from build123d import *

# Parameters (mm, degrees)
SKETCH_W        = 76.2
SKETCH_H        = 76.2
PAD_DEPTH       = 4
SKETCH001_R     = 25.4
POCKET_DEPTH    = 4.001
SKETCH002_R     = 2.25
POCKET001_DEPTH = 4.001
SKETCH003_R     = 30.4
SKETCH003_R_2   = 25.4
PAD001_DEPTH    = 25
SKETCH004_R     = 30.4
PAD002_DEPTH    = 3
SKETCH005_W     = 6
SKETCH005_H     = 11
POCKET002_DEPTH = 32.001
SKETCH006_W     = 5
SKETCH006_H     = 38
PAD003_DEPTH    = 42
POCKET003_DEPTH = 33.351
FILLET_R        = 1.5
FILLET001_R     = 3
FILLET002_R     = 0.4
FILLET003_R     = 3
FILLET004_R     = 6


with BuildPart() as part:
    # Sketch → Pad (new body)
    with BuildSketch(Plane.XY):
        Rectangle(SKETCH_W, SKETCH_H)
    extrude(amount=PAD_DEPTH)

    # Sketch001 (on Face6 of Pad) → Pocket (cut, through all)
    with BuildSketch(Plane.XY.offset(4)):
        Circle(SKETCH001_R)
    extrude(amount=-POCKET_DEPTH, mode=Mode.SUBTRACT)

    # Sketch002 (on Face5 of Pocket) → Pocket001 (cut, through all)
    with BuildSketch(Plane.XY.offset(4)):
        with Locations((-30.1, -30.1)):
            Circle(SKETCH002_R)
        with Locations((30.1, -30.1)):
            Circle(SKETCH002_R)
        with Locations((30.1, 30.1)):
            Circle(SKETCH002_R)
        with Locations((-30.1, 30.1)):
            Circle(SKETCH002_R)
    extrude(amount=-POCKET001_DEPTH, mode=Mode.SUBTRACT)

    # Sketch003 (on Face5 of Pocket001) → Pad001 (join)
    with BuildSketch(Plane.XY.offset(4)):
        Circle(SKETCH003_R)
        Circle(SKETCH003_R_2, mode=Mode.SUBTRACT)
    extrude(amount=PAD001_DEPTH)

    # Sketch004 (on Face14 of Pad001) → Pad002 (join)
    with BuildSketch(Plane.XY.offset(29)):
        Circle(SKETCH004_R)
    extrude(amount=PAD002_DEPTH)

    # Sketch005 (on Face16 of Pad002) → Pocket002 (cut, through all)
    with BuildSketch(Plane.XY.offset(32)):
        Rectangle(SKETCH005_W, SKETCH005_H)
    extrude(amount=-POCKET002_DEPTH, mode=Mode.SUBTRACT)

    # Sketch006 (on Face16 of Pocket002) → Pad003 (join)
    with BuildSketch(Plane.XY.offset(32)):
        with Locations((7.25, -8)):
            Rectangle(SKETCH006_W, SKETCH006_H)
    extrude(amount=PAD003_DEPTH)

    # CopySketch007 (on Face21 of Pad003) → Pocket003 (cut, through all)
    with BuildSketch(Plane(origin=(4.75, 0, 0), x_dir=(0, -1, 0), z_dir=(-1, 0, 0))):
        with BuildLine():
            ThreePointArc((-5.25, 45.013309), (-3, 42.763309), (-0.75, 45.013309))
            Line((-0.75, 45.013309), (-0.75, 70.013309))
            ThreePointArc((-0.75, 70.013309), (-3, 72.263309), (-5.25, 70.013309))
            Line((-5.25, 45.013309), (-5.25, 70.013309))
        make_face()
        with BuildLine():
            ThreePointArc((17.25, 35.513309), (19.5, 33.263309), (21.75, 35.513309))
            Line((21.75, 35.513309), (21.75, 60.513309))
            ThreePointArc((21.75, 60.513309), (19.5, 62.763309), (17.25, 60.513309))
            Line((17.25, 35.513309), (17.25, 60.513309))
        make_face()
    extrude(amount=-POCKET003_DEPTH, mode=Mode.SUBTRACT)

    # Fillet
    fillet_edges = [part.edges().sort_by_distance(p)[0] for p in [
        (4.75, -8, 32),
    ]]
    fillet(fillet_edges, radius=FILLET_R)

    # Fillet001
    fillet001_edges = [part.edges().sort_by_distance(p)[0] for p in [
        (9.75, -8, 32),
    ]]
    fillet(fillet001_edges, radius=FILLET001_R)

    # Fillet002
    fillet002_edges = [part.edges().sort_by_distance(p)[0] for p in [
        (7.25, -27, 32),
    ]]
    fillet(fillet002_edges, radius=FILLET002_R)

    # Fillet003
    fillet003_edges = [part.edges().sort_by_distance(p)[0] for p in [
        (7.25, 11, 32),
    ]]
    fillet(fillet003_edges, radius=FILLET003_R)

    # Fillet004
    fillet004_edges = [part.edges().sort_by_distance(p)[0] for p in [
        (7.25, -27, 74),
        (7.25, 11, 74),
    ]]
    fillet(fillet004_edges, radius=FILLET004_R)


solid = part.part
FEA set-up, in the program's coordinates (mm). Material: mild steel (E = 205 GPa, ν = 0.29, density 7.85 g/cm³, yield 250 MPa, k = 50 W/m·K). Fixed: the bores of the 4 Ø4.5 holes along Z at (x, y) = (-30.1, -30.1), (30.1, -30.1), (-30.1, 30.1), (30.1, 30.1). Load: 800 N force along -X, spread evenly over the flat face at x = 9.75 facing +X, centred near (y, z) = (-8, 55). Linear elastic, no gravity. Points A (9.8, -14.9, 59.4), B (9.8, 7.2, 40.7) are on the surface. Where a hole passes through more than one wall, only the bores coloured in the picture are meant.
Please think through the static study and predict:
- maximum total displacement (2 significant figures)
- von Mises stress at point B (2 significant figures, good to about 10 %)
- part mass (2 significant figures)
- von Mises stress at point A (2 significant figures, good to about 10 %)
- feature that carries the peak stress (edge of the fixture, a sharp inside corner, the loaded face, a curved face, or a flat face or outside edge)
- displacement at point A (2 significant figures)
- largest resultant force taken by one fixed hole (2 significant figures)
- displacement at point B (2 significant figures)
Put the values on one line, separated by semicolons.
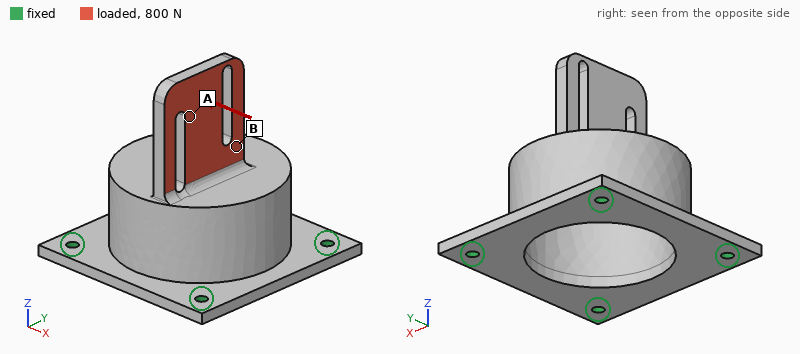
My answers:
0.19 mm; 78 MPa; 410 g; 24 MPa; a curved face; 0.12 mm; 470 N; 0.032 mm
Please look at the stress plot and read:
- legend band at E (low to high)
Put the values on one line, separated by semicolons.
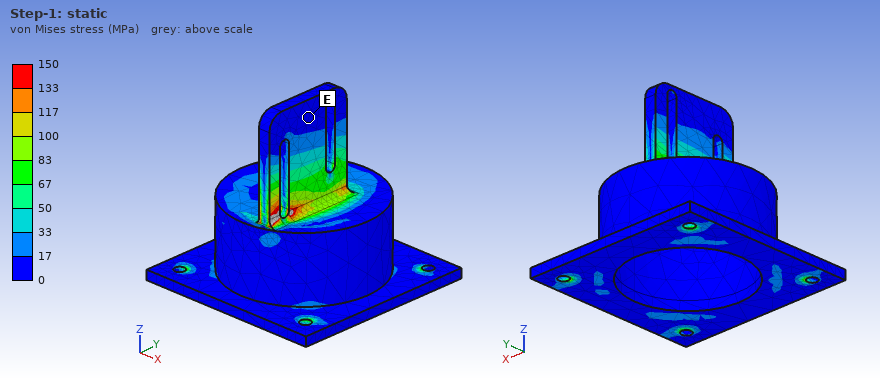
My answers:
0 to 17 MPa
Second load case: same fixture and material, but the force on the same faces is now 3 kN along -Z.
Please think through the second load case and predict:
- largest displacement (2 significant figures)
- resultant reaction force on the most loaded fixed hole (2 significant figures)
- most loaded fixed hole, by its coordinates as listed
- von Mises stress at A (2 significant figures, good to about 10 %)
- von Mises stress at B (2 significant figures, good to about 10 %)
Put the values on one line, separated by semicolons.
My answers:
81 µm; 1.3 kN; (30.1, -30.1); 25 MPa; 60 MPa
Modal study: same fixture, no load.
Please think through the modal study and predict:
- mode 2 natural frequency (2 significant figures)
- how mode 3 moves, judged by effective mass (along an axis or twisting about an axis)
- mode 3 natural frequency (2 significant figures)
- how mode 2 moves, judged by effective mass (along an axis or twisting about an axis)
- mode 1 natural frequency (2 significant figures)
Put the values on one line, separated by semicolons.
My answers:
3200 Hz; along Z; 4200 Hz; along Y; 1800 Hz
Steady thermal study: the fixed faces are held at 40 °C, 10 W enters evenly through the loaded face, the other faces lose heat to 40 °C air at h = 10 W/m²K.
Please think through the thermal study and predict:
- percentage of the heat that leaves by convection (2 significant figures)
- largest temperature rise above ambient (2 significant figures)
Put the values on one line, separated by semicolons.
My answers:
27 %; 47 K
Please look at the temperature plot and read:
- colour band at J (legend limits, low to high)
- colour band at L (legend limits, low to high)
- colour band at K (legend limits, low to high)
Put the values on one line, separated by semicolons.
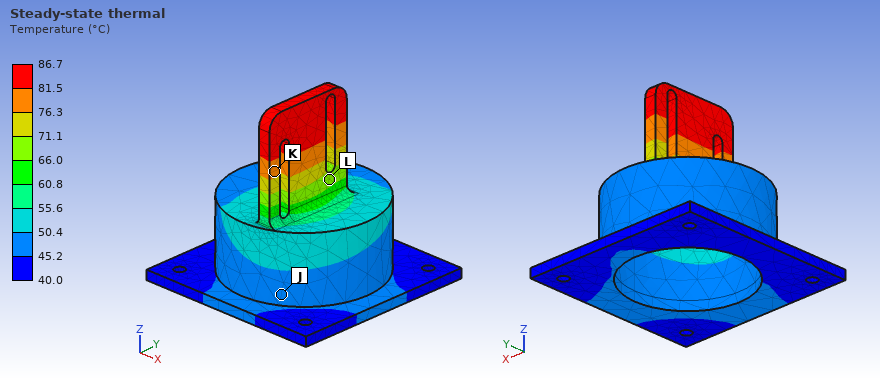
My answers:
45.2 to 50.4 °C; 66.0 to 71.1 °C; 76.3 to 81.5 °C
